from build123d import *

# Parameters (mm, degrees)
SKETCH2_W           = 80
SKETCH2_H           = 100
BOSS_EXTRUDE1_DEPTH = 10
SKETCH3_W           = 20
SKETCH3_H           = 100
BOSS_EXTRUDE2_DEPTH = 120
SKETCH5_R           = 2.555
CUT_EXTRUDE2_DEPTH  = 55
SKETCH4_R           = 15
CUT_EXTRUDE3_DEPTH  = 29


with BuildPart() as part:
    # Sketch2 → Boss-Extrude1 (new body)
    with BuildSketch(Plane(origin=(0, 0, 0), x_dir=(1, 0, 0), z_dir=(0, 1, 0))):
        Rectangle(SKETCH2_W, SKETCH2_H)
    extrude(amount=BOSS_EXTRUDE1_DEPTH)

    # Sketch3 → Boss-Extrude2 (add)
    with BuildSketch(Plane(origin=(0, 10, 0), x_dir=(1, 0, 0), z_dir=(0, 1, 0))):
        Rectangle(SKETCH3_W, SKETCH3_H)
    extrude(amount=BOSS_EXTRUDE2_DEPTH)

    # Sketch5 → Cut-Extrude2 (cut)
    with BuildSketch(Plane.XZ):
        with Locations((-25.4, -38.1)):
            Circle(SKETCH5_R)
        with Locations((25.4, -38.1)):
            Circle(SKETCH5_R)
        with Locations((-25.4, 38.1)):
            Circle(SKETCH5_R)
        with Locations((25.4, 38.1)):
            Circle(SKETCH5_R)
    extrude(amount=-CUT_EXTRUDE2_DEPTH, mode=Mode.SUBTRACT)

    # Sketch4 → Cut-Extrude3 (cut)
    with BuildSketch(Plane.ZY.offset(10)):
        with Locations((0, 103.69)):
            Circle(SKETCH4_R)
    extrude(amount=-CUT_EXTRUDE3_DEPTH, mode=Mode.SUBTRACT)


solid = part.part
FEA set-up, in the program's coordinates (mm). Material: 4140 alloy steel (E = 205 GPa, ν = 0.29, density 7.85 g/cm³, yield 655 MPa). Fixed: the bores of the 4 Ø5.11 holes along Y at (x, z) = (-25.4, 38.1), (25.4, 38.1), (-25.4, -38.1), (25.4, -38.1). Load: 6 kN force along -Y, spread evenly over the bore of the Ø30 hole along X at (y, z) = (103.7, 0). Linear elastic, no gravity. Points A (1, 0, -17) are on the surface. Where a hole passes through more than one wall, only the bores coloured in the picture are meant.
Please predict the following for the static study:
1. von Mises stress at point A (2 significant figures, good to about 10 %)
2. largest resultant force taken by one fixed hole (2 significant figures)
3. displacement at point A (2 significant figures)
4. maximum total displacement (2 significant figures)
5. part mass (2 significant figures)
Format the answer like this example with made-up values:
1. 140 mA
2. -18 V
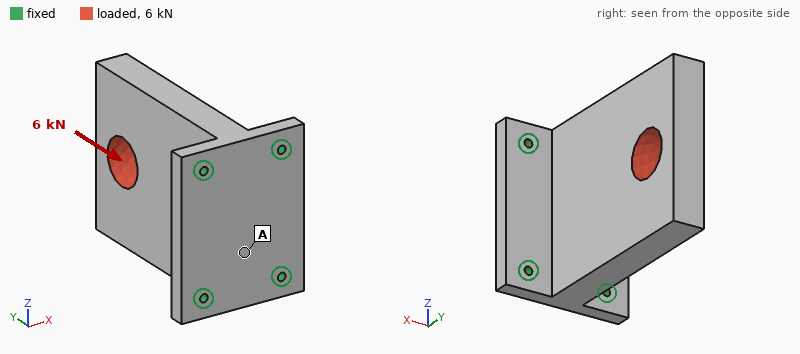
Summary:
1. 6.7 MPa
2. 1.5 kN
3. 3.9 µm
4. 6.6 µm
5. 2.4 kg
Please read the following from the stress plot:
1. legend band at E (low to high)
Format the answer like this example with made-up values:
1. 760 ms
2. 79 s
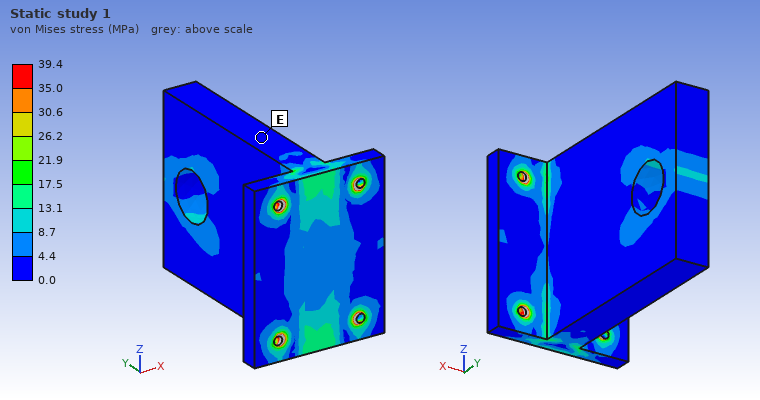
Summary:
1. 0.0 to 4.4 MPa
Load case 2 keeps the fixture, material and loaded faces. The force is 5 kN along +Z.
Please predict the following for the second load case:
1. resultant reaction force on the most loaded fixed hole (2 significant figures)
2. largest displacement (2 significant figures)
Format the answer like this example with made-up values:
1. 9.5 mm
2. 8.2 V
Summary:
1. 3.6 kN
2. 40 µm
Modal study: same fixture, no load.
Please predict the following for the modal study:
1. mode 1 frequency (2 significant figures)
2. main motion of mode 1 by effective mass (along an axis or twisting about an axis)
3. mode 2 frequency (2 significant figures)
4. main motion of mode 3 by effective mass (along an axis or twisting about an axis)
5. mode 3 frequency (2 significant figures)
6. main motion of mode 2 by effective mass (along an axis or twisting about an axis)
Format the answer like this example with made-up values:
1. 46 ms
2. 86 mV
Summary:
1. 890 Hz
2. along X
3. 2000 Hz
4. twisting about Y
5. 2600 Hz
6. along Z
